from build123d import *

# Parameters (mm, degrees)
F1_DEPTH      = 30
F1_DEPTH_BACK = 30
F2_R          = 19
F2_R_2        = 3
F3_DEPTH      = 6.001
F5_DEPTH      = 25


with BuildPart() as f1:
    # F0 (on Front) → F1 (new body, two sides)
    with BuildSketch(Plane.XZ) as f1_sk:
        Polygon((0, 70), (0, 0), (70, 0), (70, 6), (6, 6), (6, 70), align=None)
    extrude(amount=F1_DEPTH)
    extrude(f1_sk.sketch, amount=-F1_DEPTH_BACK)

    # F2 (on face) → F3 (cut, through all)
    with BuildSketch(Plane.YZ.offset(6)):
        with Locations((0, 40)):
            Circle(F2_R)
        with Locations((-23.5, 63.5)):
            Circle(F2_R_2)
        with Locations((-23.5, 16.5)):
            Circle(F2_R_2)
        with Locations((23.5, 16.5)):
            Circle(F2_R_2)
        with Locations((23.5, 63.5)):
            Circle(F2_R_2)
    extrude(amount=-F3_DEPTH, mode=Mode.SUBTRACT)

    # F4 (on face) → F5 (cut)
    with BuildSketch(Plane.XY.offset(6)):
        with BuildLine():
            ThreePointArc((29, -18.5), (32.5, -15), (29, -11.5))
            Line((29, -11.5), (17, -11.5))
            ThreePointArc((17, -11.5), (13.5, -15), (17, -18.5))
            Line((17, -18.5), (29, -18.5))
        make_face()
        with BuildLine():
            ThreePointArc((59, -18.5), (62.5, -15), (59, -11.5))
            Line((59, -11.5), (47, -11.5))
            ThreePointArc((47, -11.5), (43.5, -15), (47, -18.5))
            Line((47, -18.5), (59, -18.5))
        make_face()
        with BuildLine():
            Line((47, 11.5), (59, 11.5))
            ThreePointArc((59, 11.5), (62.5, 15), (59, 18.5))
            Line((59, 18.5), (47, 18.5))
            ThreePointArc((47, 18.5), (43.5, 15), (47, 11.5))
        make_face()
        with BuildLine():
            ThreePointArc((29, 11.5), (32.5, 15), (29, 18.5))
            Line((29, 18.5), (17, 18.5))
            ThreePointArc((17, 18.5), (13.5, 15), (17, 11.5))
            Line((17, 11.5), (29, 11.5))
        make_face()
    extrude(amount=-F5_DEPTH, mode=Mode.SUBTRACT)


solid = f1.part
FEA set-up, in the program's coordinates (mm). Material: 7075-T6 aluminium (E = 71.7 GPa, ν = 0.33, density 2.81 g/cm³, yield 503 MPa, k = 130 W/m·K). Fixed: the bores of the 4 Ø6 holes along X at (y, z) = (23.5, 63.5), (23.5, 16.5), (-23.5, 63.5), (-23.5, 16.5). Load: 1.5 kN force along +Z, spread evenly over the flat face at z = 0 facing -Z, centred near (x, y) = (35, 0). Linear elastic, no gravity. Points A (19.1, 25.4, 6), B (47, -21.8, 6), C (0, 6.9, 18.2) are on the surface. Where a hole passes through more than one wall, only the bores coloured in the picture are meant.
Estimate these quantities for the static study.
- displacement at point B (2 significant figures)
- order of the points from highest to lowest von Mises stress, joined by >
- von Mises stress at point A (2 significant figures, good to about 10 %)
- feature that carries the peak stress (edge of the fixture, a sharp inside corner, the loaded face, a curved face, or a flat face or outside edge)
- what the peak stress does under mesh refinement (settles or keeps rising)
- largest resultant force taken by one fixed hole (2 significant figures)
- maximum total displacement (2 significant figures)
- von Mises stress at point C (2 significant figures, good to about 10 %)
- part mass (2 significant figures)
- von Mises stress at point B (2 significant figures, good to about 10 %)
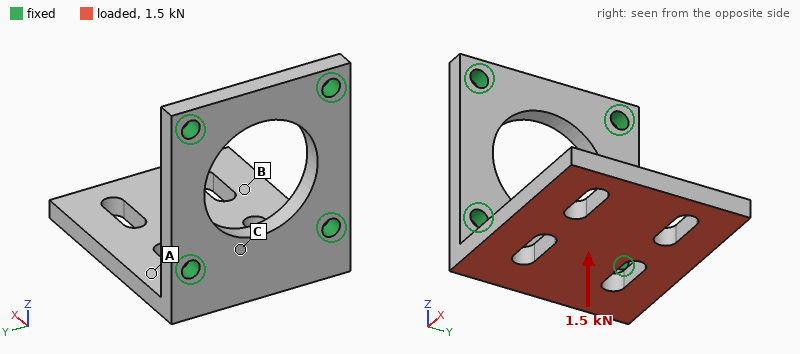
0.75 mm
A > C > B
91 MPa
edge of the fixture
keeps rising
790 N
1.3 mm
57 MPa
110 g
21 MPa
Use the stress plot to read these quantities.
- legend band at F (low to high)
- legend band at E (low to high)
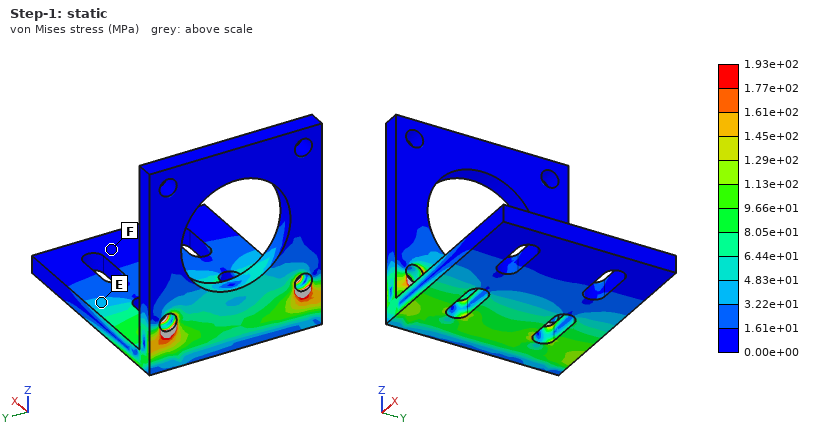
0.00e+00 to 1.61e+01 MPa
3.22e+01 to 4.83e+01 MPa
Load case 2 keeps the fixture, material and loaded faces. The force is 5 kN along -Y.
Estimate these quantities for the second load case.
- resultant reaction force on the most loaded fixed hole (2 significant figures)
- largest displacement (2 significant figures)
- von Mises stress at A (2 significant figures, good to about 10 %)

4.4 kN
0.24 mm
69 MPa
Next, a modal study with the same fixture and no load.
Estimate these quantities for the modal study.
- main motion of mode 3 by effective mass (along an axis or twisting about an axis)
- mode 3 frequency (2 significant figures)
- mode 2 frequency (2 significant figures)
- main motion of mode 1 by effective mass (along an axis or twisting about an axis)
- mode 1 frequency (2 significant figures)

along Y
3500 Hz
2400 Hz
along Z
840 Hz
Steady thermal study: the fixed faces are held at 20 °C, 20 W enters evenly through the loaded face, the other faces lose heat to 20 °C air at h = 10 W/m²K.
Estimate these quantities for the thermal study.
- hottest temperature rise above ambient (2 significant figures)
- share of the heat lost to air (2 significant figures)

21 K
5.2 %
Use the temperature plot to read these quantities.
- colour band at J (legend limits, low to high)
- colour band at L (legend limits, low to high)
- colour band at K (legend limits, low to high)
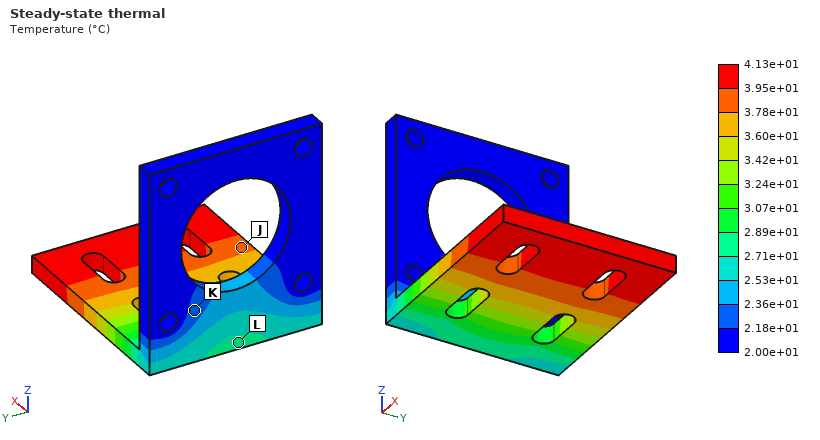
3.78e+01 to 3.95e+01 °C
2.71e+01 to 2.89e+01 °C
2.18e+01 to 2.36e+01 °C
